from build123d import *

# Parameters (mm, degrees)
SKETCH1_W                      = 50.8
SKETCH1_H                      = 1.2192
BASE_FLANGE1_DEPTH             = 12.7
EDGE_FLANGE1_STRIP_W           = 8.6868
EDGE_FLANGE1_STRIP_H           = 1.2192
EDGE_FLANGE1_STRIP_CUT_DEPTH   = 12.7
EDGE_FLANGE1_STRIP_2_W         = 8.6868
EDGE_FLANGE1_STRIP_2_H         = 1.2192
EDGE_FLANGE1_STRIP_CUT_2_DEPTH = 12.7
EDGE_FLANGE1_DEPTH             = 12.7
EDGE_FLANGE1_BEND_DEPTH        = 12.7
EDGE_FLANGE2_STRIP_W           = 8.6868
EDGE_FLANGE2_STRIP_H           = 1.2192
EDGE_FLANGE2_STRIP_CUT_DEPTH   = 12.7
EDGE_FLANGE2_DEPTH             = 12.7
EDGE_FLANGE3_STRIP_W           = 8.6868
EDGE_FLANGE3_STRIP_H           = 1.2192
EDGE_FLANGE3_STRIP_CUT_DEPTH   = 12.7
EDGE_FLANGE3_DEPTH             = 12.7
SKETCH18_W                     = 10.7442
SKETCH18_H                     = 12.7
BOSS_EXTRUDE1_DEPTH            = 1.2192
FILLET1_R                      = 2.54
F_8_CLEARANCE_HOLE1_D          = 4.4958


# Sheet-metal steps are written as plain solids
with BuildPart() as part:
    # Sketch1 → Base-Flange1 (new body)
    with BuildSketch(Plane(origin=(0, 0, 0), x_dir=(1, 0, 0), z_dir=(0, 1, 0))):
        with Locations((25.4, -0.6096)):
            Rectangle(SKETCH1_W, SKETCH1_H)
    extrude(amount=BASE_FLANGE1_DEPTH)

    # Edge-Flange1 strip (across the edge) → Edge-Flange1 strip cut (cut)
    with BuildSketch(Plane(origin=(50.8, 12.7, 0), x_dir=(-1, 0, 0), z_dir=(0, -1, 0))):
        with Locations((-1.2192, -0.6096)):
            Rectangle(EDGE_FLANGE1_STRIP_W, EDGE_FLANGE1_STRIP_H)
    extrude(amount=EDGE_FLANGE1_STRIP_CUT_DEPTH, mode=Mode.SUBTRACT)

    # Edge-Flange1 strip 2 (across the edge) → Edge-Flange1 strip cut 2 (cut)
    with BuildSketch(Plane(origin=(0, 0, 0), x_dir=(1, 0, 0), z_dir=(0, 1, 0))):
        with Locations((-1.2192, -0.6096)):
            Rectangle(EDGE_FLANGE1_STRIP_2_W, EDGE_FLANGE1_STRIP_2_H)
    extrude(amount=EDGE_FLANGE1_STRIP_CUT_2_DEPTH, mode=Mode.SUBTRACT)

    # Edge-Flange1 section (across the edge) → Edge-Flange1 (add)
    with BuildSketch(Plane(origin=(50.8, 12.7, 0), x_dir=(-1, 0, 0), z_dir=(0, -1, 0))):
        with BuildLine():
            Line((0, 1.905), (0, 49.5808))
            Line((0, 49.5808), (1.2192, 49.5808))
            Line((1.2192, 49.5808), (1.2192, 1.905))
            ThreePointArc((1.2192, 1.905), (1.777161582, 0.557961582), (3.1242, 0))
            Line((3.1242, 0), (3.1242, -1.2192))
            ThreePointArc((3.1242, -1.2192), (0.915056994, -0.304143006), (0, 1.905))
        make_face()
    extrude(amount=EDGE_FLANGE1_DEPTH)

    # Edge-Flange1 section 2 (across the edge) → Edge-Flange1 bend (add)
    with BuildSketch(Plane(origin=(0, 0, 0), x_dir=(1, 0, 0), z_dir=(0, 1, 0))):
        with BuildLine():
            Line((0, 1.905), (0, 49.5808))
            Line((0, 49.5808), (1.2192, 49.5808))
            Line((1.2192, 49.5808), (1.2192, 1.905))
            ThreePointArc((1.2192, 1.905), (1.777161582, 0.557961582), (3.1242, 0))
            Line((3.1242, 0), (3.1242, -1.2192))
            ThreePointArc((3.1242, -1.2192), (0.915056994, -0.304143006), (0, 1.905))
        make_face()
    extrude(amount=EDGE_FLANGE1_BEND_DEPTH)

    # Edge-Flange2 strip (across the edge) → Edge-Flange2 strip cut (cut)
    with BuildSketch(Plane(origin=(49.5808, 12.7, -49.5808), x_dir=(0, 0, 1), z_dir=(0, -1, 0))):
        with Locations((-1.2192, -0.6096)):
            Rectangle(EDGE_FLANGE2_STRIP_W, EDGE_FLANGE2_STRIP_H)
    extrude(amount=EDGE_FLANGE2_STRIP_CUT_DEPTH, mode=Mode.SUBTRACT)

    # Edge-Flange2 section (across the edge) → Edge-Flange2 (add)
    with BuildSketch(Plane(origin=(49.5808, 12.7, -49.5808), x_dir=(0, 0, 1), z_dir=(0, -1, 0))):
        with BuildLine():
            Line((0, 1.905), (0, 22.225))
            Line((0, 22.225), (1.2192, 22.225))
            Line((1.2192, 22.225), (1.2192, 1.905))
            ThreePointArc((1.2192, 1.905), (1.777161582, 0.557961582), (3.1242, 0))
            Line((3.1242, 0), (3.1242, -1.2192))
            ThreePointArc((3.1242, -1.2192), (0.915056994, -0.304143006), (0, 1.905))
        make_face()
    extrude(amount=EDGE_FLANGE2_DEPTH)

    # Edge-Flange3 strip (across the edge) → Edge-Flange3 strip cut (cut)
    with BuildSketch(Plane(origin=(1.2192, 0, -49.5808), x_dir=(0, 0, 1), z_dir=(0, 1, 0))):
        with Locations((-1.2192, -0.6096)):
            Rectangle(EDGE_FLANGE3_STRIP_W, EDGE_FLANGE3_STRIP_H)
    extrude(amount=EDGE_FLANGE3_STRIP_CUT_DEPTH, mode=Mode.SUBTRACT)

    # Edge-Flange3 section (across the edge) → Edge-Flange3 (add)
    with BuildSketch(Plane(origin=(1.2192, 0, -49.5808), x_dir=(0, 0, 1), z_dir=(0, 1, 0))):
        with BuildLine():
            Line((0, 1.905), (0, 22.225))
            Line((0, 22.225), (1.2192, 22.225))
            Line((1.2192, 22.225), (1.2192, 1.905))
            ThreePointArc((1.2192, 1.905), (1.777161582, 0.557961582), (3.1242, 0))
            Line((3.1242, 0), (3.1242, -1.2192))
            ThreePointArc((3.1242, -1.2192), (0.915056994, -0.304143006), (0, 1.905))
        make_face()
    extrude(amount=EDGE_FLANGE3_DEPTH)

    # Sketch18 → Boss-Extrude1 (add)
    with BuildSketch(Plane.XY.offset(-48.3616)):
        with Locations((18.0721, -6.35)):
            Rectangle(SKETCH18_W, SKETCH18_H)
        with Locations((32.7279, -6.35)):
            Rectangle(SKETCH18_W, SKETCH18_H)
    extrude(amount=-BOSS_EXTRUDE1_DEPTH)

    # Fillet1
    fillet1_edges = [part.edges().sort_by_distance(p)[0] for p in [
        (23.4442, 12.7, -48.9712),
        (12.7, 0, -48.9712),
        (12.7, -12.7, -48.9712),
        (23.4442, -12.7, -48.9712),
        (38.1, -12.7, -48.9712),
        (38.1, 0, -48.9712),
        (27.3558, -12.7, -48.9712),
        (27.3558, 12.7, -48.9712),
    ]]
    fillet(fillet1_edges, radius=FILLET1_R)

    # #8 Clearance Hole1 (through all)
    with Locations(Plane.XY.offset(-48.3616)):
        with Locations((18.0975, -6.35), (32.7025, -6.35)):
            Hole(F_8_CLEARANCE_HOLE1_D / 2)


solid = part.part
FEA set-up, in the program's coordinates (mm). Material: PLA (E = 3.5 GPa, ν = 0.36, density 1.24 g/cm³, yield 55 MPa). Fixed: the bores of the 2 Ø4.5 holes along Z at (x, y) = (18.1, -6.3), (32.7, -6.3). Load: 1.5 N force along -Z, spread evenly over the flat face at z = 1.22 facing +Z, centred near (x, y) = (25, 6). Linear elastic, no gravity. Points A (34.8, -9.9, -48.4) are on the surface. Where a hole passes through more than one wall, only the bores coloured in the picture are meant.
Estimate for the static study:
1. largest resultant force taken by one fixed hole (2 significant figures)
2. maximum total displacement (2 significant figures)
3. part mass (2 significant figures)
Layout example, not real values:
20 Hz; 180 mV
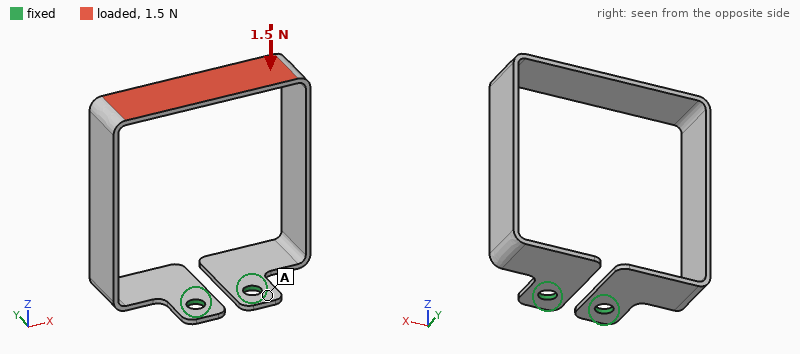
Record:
0.75 N; 0.74 mm; 4.0 g
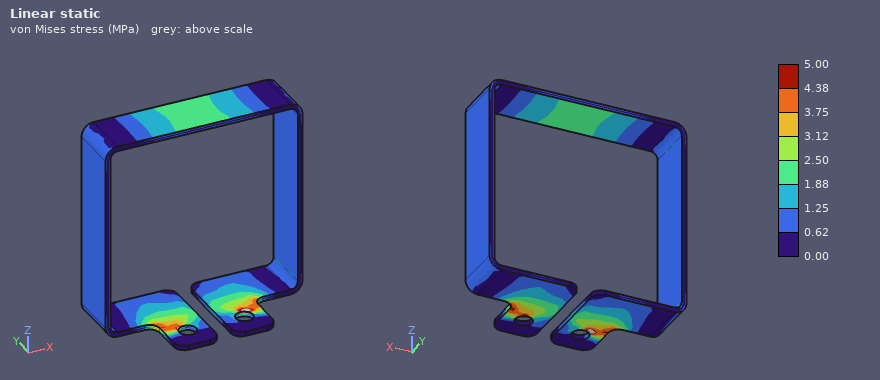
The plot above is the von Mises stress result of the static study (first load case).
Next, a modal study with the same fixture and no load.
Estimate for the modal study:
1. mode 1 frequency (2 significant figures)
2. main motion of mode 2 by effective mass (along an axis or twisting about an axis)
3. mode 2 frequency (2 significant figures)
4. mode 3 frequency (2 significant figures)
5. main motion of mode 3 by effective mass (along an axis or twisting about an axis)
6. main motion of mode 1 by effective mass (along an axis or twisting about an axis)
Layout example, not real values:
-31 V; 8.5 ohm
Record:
70 Hz; along X; 73 Hz; 190 Hz; twisting about Z; along Y
